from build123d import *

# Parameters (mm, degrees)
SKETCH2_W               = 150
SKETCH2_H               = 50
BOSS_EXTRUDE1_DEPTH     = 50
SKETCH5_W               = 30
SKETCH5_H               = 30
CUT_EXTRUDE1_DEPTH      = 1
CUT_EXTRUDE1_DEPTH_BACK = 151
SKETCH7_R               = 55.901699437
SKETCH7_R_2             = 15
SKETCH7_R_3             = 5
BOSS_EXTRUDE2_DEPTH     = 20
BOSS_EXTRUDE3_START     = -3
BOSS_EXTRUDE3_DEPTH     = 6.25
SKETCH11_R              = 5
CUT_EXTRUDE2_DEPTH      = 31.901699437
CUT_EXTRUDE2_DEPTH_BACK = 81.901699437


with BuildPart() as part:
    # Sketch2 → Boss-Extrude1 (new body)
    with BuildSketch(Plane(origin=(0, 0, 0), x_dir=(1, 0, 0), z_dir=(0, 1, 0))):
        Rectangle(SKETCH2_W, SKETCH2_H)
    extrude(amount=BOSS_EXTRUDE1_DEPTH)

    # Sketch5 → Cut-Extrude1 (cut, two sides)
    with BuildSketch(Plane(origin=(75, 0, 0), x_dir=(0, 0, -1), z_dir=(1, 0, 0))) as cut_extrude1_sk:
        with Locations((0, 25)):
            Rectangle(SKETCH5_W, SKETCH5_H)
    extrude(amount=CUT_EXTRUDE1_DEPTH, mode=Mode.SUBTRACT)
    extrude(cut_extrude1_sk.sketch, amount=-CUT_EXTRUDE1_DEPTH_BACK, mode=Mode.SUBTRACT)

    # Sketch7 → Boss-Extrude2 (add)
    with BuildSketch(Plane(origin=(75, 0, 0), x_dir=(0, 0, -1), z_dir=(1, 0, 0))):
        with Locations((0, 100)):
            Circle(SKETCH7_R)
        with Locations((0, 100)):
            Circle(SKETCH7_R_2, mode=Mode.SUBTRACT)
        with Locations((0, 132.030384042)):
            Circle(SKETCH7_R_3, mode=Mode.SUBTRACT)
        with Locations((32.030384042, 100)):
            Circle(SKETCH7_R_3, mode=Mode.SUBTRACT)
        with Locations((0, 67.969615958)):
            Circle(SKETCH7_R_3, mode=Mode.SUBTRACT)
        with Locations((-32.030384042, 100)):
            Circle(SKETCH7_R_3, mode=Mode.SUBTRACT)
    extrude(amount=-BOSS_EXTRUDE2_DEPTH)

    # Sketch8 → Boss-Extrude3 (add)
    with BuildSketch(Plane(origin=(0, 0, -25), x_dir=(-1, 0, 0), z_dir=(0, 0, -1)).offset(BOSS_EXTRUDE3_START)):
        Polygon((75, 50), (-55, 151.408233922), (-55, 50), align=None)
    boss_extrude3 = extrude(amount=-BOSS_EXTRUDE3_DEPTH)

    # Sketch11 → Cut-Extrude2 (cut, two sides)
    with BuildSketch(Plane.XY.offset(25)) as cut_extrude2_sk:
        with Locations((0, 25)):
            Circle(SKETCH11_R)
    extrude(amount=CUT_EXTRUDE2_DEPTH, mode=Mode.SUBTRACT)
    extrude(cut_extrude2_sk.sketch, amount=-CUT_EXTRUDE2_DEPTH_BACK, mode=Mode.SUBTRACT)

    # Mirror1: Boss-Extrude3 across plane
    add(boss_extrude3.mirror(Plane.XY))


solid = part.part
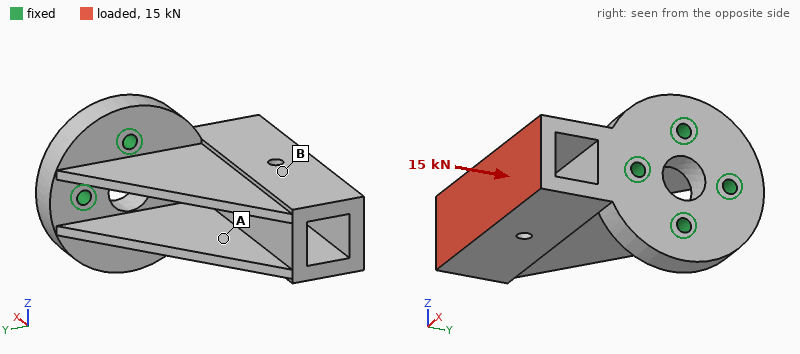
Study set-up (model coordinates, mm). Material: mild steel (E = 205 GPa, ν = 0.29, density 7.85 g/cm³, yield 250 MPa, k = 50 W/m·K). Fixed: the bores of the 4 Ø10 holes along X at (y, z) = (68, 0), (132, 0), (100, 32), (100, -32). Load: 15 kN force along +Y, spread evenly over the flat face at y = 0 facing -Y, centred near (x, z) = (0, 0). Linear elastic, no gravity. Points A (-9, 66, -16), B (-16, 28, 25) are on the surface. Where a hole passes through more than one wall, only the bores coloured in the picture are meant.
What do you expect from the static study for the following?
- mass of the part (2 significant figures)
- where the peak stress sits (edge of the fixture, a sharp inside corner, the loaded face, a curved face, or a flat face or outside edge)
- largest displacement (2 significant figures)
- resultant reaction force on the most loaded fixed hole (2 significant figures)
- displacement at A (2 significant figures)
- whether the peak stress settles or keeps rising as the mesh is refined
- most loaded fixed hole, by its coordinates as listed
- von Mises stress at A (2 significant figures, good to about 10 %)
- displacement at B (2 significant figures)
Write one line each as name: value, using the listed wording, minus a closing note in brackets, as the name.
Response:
mass of the part: 3.9 kg
where the peak stress sits: edge of the fixture
largest displacement: 57 µm
resultant reaction force on the most loaded fixed hole: 13 kN
displacement at A: 24 µm
whether the peak stress settles or keeps rising as the mesh is refined: keeps rising
most loaded fixed hole, by its coordinates as listed: (68, 0)
von Mises stress at A: 16 MPa
displacement at B: 33 µm
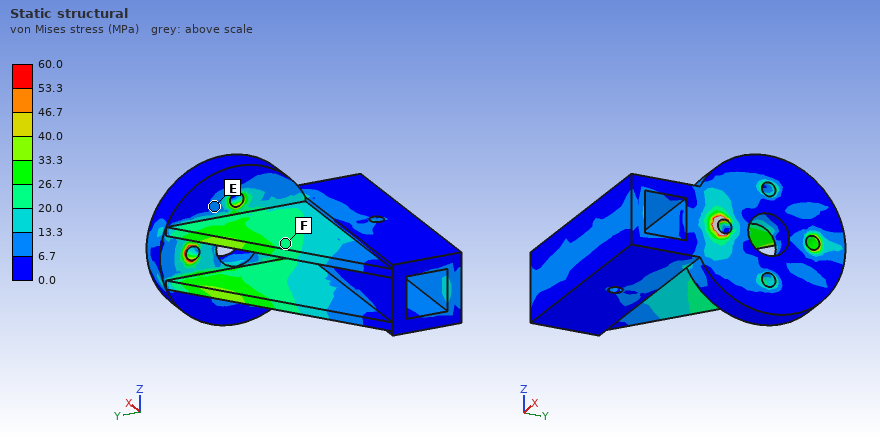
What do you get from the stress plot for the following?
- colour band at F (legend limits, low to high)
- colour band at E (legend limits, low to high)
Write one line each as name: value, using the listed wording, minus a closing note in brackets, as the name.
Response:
colour band at F: 20.0 to 26.7 MPa
colour band at E: 6.7 to 13.3 MPa
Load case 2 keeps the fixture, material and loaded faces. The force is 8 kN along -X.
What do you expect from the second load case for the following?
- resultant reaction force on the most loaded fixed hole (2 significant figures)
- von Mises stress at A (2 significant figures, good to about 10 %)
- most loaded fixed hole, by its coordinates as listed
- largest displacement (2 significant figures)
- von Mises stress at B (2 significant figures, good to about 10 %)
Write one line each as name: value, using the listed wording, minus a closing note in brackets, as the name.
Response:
resultant reaction force on the most loaded fixed hole: 13 kN
von Mises stress at A: 6.7 MPa
most loaded fixed hole, by its coordinates as listed: (68, 0)
largest displacement: 40 µm
von Mises stress at B: 6.2 MPa
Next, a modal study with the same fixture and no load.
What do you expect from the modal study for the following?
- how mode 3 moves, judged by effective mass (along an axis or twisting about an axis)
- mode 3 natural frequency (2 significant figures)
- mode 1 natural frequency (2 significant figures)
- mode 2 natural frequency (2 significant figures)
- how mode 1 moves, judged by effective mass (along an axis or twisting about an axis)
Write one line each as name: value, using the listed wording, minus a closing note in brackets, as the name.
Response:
how mode 3 moves, judged by effective mass: twisting about X
mode 3 natural frequency: 2600 Hz
mode 1 natural frequency: 1100 Hz
mode 2 natural frequency: 1900 Hz
how mode 1 moves, judged by effective mass: along Z
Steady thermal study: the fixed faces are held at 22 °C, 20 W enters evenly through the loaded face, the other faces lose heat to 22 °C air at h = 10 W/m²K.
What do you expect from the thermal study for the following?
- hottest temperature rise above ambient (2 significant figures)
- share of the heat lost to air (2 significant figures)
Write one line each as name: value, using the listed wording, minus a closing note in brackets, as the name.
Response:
hottest temperature rise above ambient: 16 K
share of the heat lost to air: 31 %
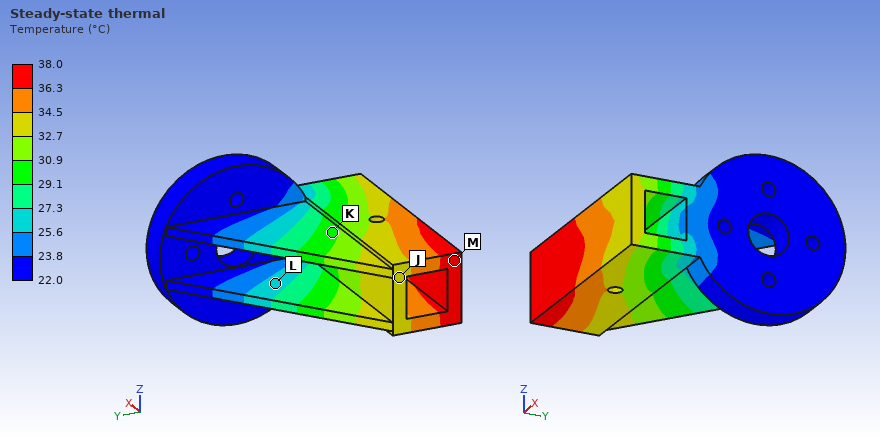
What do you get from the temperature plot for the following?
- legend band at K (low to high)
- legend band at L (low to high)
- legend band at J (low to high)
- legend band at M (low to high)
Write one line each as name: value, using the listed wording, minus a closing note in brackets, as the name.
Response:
legend band at K: 29.1 to 30.9 °C
legend band at L: 25.6 to 27.3 °C
legend band at J: 32.7 to 34.5 °C
legend band at M: 36.3 to 38.0 °C
